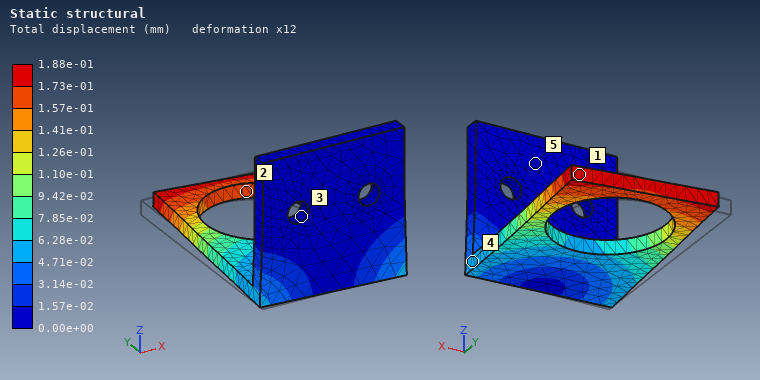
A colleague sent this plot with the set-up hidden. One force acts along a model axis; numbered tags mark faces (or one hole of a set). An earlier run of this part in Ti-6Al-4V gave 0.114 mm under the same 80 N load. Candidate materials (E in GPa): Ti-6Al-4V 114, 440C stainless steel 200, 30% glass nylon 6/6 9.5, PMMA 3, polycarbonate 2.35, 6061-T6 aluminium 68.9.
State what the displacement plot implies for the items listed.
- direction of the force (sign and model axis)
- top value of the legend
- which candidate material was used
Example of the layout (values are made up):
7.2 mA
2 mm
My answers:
+X
1.88e-01 mm
6061-T6 aluminium
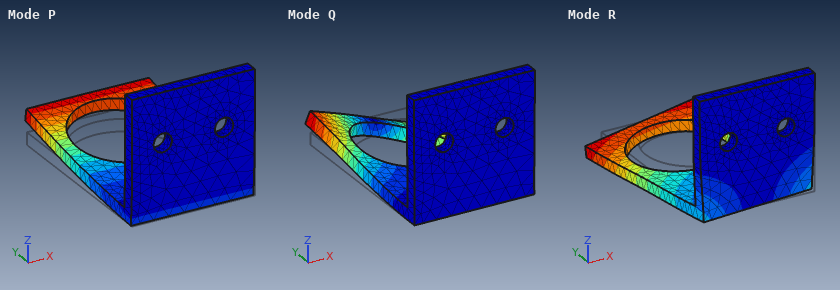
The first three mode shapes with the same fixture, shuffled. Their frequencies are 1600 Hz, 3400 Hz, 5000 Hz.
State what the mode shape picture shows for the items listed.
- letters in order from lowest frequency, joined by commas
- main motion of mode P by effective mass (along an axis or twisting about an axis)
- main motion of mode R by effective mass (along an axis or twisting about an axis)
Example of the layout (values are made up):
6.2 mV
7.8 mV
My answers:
P, R, Q
along Z
along X
